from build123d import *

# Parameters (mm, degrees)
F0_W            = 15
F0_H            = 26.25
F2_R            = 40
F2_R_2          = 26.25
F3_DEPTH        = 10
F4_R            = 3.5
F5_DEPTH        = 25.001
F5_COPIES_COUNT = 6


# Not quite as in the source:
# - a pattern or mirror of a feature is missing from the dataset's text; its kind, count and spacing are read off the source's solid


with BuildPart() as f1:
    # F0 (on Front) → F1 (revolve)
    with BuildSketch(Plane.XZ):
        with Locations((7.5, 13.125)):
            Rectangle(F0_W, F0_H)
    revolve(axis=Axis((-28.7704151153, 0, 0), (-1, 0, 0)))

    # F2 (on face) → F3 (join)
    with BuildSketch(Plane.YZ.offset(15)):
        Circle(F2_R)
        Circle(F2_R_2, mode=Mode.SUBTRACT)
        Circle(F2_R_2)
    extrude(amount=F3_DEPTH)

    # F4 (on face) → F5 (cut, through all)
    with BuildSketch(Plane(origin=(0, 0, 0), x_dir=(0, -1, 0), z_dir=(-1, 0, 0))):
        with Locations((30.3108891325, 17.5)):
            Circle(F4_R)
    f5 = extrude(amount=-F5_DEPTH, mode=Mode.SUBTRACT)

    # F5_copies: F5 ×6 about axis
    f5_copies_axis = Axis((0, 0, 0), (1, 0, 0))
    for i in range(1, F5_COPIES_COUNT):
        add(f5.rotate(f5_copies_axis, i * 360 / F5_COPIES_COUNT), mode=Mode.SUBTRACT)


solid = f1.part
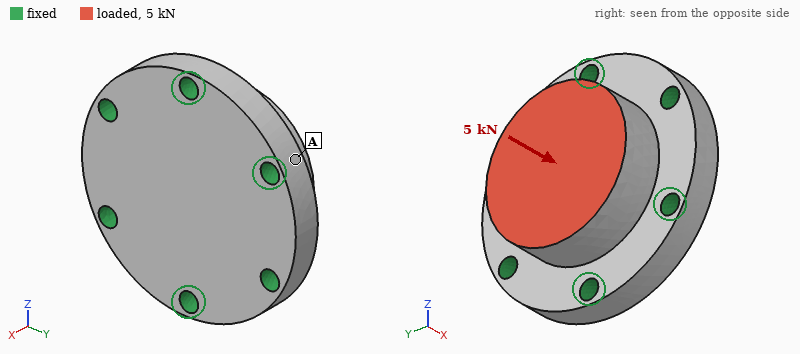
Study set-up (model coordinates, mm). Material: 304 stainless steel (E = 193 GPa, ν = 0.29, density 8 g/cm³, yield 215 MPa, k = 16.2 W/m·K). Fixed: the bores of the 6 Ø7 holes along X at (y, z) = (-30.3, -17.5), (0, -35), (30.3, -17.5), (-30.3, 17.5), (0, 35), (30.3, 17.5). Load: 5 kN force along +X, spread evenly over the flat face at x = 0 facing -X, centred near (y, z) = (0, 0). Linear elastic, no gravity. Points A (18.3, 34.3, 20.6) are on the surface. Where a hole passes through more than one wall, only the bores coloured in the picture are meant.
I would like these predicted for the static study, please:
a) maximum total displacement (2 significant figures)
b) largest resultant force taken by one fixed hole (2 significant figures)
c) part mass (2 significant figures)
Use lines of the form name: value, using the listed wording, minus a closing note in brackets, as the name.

maximum total displacement: 1.4 µm
largest resultant force taken by one fixed hole: 890 N
part mass: 640 g
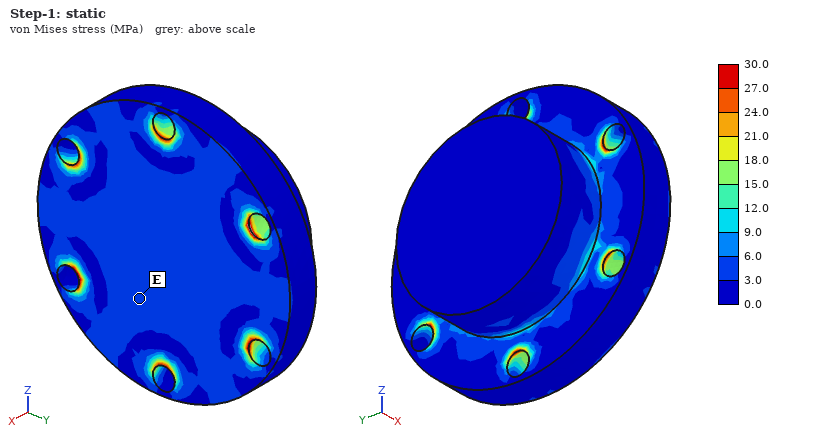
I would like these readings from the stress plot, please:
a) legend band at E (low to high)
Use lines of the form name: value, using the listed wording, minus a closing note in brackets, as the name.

legend band at E: 3.0 to 6.0 MPa
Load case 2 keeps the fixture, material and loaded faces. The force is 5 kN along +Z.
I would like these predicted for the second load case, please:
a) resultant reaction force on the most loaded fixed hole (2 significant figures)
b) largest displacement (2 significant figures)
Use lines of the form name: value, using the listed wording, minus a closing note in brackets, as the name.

resultant reaction force on the most loaded fixed hole: 1.6 kN
largest displacement: 2.3 µm
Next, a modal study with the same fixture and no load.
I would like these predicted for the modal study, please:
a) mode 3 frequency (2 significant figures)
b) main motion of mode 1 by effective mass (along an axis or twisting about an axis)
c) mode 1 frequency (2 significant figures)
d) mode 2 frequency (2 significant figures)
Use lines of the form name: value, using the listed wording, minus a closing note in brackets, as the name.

mode 3 frequency: 19 kHz
main motion of mode 1 by effective mass: along X
mode 1 frequency: 15 kHz
mode 2 frequency: 19 kHz
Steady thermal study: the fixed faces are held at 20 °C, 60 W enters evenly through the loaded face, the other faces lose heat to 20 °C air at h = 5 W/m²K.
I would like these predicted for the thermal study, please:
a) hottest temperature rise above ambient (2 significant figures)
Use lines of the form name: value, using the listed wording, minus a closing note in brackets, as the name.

hottest temperature rise above ambient: 64 K
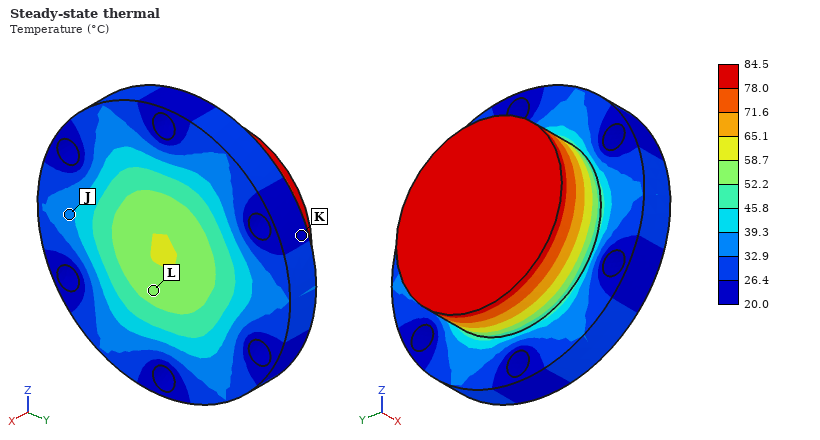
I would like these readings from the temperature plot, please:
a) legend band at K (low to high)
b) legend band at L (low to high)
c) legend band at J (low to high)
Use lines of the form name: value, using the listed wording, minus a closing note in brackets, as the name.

legend band at K: 20.0 to 26.4 °C
legend band at L: 52.2 to 58.7 °C
legend band at J: 32.9 to 39.3 °C
